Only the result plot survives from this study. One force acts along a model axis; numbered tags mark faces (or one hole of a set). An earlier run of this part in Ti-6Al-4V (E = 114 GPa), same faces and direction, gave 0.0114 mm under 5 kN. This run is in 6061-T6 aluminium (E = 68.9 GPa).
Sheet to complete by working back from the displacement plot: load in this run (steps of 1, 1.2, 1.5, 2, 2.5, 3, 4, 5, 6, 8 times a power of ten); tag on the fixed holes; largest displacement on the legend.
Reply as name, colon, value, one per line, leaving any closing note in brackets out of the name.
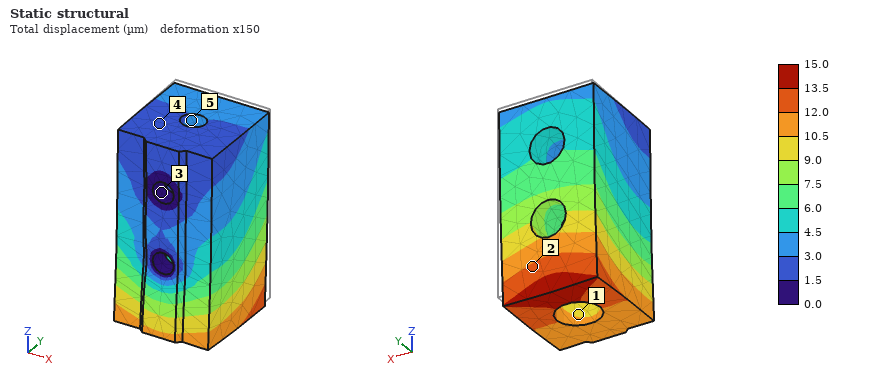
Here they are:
load in this run: 4 kN
tag on the fixed holes: 3
largest displacement on the legend: 15.0 µm
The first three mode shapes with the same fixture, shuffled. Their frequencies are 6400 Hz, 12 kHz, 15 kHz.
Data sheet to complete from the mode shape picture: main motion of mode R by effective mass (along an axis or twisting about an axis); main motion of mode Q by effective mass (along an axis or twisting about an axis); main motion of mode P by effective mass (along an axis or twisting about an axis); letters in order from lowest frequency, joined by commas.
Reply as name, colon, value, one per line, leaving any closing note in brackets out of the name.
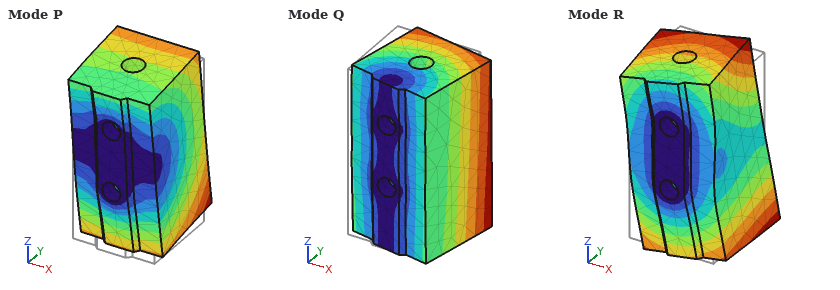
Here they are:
main motion of mode R by effective mass: twisting about Y
main motion of mode Q by effective mass: along X
main motion of mode P by effective mass: along Z
letters in order from lowest frequency, joined by commas: Q, P, R
